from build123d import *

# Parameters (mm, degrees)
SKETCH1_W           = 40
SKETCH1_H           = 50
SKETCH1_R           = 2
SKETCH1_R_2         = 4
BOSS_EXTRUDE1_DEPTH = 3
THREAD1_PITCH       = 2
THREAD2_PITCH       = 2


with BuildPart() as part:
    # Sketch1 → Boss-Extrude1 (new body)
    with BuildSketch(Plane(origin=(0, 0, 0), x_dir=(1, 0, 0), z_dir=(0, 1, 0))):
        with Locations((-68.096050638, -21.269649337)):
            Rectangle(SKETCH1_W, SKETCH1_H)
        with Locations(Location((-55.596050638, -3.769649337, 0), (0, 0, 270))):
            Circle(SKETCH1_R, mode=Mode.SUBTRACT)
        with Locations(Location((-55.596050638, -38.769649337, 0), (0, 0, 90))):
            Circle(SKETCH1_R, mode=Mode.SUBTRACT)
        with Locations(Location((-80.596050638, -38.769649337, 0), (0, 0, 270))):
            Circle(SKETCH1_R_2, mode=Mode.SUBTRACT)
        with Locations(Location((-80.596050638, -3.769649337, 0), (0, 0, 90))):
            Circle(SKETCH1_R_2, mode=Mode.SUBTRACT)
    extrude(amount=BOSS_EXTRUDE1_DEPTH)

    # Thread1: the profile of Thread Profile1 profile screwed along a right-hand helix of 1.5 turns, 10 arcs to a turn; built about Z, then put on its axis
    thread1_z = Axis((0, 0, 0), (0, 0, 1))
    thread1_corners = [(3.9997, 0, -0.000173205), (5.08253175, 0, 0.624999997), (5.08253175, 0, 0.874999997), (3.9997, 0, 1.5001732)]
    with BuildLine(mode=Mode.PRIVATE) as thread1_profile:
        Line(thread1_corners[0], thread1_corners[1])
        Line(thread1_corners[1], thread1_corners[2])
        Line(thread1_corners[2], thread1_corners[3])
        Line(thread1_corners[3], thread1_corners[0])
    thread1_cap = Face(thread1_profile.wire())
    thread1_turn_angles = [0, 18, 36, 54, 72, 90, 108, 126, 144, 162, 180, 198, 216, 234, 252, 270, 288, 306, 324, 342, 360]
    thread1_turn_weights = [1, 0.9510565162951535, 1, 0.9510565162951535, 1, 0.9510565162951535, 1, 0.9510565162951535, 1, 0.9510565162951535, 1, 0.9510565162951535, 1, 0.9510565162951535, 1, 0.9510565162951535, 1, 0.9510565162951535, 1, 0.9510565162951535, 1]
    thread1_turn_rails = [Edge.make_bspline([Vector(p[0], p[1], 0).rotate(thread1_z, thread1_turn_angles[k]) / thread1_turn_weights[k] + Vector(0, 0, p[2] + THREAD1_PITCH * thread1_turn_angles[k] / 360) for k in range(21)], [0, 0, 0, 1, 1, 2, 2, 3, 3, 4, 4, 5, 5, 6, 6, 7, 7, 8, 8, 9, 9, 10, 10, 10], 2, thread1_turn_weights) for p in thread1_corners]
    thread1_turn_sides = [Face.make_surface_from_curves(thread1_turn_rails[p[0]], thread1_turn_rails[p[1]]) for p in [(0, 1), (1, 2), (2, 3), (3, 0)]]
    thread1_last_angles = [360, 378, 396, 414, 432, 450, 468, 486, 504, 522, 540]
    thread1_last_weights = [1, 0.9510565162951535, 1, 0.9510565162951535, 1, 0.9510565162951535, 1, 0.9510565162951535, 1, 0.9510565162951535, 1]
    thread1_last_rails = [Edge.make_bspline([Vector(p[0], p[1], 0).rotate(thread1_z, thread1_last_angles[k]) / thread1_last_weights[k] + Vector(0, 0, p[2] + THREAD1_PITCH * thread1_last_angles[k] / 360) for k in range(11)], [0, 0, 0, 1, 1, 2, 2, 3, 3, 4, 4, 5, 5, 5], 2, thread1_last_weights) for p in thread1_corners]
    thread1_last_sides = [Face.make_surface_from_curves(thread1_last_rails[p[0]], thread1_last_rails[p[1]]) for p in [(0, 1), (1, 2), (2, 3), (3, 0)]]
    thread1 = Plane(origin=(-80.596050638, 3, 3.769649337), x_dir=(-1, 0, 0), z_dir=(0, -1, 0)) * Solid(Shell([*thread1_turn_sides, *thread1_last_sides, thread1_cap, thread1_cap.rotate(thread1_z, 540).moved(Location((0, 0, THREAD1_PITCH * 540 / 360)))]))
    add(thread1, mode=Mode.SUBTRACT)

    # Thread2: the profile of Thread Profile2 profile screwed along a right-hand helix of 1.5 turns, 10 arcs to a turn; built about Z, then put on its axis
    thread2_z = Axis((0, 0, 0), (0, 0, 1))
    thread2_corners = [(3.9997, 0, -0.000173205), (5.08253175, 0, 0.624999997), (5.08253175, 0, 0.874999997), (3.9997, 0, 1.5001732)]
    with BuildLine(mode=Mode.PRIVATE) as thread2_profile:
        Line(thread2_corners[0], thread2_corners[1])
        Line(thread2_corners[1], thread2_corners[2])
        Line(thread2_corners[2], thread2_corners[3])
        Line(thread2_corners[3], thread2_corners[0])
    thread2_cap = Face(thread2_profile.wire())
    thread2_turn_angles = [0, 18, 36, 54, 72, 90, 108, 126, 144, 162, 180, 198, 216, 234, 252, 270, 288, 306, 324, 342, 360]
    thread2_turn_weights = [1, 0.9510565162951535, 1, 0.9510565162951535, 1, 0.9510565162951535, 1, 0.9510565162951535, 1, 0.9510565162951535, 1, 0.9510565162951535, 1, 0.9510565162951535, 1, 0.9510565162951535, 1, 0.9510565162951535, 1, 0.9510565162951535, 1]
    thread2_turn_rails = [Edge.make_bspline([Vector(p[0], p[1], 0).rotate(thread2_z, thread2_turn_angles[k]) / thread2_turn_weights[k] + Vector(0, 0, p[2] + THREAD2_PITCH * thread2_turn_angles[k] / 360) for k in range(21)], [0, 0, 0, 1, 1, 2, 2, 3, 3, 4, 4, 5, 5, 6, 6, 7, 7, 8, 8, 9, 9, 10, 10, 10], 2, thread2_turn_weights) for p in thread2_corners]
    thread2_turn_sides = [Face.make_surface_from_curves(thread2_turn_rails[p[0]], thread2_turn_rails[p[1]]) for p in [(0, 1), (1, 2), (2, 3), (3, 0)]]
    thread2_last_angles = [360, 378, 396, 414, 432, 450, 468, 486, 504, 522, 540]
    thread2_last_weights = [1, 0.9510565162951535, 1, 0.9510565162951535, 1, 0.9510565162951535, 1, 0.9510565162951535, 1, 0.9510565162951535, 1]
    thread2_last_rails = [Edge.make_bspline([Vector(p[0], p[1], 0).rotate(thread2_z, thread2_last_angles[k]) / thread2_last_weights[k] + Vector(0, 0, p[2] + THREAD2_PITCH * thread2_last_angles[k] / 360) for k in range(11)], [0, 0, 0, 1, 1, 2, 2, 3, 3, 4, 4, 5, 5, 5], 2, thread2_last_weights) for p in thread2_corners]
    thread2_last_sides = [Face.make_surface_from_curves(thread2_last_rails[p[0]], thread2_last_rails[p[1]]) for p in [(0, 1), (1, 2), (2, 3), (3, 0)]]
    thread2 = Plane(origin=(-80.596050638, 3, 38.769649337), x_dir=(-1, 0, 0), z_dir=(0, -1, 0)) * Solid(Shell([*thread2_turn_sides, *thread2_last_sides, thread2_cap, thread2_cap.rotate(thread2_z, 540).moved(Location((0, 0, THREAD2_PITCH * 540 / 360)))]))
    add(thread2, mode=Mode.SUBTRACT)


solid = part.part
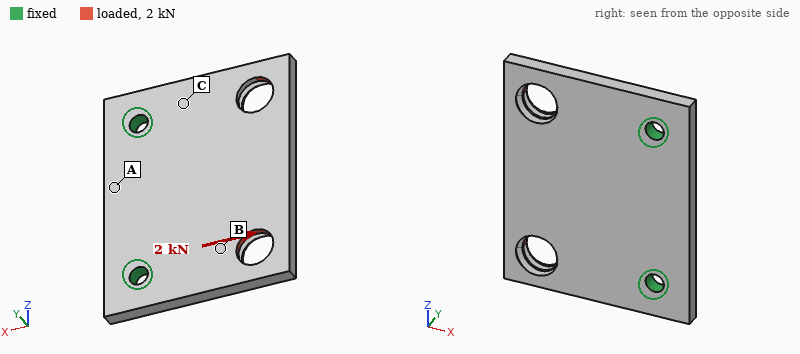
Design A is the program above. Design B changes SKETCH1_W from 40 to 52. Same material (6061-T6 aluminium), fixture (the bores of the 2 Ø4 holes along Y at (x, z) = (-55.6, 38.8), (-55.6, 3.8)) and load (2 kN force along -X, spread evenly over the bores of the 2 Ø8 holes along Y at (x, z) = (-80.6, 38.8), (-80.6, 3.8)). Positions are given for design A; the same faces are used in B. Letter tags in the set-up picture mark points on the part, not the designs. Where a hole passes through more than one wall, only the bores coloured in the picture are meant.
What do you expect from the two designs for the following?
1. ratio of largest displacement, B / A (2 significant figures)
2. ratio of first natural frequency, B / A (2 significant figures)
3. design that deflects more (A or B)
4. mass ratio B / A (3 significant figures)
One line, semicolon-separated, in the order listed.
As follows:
1.2; 0.70; B; 1.32
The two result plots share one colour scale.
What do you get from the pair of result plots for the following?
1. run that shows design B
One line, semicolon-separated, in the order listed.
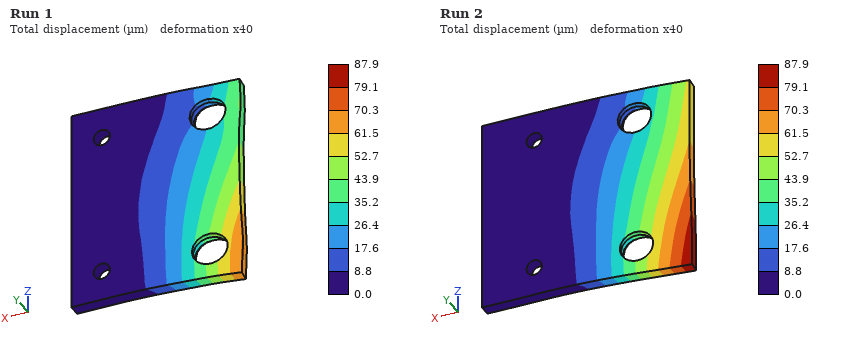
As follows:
Run 2
